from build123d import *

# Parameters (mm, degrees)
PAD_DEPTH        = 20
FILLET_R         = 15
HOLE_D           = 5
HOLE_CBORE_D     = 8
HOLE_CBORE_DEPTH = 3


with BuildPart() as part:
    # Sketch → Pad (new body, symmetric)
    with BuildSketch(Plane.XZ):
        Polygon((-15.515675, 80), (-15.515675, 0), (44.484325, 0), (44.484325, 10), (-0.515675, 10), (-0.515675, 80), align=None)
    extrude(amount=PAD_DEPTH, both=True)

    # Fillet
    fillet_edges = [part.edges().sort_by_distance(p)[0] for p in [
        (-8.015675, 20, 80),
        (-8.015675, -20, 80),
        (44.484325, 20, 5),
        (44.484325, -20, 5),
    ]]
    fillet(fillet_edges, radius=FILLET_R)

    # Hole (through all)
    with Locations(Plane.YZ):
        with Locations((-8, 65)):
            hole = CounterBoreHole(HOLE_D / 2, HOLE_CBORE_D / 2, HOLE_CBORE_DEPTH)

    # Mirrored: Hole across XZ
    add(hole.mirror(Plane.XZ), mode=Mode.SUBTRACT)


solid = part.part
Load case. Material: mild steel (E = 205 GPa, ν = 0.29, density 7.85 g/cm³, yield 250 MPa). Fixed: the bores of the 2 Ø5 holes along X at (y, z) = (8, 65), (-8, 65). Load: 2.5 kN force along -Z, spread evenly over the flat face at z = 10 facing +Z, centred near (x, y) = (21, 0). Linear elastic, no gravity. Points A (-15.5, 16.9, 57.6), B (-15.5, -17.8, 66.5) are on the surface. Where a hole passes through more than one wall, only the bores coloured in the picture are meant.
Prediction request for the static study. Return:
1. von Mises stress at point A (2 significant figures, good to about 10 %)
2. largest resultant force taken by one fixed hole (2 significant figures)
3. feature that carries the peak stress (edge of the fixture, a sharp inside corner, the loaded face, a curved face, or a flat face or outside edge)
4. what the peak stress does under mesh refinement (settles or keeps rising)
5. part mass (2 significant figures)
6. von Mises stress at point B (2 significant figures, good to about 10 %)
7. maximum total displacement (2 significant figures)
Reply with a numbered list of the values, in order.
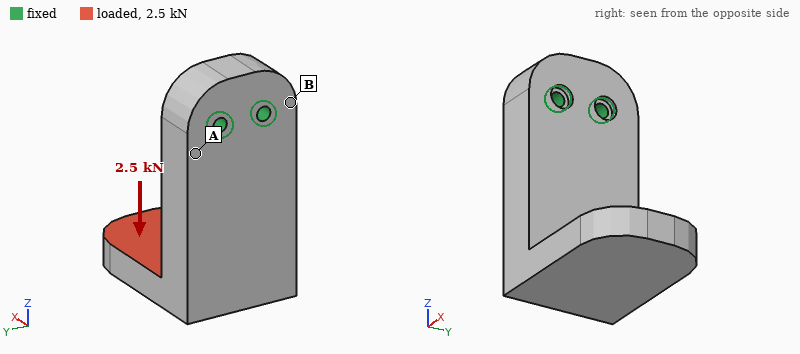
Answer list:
1. 38 MPa
2. 1.3 kN
3. edge of the fixture
4. keeps rising
5. 490 g
6. 18 MPa
7. 0.18 mm
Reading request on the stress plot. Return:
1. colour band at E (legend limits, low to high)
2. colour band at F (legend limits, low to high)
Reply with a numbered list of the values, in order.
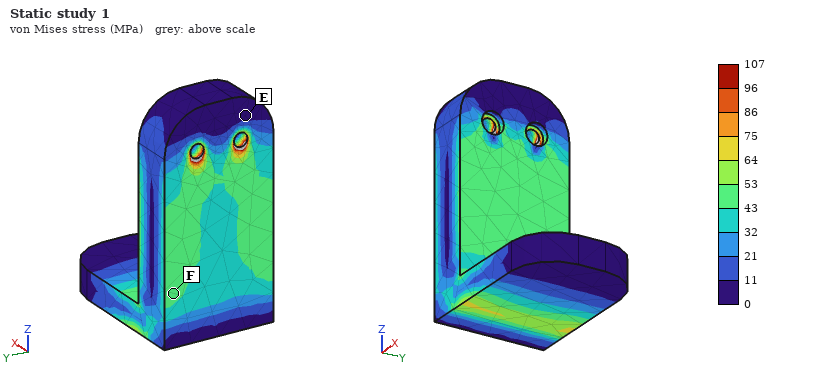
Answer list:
1. 0 to 11 MPa
2. 43 to 53 MPa
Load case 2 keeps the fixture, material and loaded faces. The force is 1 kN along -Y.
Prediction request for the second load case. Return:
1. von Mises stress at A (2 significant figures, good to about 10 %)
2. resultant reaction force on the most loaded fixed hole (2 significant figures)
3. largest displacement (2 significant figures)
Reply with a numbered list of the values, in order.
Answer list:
1. 17 MPa
2. 3.1 kN
3. 40 µm
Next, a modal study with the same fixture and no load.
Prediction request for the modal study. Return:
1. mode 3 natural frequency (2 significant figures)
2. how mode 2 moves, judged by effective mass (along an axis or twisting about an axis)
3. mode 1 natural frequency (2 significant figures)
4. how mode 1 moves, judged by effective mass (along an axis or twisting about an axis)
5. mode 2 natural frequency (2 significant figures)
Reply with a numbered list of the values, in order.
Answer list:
1. 3500 Hz
2. along Y
3. 1400 Hz
4. along X
5. 2400 Hz
